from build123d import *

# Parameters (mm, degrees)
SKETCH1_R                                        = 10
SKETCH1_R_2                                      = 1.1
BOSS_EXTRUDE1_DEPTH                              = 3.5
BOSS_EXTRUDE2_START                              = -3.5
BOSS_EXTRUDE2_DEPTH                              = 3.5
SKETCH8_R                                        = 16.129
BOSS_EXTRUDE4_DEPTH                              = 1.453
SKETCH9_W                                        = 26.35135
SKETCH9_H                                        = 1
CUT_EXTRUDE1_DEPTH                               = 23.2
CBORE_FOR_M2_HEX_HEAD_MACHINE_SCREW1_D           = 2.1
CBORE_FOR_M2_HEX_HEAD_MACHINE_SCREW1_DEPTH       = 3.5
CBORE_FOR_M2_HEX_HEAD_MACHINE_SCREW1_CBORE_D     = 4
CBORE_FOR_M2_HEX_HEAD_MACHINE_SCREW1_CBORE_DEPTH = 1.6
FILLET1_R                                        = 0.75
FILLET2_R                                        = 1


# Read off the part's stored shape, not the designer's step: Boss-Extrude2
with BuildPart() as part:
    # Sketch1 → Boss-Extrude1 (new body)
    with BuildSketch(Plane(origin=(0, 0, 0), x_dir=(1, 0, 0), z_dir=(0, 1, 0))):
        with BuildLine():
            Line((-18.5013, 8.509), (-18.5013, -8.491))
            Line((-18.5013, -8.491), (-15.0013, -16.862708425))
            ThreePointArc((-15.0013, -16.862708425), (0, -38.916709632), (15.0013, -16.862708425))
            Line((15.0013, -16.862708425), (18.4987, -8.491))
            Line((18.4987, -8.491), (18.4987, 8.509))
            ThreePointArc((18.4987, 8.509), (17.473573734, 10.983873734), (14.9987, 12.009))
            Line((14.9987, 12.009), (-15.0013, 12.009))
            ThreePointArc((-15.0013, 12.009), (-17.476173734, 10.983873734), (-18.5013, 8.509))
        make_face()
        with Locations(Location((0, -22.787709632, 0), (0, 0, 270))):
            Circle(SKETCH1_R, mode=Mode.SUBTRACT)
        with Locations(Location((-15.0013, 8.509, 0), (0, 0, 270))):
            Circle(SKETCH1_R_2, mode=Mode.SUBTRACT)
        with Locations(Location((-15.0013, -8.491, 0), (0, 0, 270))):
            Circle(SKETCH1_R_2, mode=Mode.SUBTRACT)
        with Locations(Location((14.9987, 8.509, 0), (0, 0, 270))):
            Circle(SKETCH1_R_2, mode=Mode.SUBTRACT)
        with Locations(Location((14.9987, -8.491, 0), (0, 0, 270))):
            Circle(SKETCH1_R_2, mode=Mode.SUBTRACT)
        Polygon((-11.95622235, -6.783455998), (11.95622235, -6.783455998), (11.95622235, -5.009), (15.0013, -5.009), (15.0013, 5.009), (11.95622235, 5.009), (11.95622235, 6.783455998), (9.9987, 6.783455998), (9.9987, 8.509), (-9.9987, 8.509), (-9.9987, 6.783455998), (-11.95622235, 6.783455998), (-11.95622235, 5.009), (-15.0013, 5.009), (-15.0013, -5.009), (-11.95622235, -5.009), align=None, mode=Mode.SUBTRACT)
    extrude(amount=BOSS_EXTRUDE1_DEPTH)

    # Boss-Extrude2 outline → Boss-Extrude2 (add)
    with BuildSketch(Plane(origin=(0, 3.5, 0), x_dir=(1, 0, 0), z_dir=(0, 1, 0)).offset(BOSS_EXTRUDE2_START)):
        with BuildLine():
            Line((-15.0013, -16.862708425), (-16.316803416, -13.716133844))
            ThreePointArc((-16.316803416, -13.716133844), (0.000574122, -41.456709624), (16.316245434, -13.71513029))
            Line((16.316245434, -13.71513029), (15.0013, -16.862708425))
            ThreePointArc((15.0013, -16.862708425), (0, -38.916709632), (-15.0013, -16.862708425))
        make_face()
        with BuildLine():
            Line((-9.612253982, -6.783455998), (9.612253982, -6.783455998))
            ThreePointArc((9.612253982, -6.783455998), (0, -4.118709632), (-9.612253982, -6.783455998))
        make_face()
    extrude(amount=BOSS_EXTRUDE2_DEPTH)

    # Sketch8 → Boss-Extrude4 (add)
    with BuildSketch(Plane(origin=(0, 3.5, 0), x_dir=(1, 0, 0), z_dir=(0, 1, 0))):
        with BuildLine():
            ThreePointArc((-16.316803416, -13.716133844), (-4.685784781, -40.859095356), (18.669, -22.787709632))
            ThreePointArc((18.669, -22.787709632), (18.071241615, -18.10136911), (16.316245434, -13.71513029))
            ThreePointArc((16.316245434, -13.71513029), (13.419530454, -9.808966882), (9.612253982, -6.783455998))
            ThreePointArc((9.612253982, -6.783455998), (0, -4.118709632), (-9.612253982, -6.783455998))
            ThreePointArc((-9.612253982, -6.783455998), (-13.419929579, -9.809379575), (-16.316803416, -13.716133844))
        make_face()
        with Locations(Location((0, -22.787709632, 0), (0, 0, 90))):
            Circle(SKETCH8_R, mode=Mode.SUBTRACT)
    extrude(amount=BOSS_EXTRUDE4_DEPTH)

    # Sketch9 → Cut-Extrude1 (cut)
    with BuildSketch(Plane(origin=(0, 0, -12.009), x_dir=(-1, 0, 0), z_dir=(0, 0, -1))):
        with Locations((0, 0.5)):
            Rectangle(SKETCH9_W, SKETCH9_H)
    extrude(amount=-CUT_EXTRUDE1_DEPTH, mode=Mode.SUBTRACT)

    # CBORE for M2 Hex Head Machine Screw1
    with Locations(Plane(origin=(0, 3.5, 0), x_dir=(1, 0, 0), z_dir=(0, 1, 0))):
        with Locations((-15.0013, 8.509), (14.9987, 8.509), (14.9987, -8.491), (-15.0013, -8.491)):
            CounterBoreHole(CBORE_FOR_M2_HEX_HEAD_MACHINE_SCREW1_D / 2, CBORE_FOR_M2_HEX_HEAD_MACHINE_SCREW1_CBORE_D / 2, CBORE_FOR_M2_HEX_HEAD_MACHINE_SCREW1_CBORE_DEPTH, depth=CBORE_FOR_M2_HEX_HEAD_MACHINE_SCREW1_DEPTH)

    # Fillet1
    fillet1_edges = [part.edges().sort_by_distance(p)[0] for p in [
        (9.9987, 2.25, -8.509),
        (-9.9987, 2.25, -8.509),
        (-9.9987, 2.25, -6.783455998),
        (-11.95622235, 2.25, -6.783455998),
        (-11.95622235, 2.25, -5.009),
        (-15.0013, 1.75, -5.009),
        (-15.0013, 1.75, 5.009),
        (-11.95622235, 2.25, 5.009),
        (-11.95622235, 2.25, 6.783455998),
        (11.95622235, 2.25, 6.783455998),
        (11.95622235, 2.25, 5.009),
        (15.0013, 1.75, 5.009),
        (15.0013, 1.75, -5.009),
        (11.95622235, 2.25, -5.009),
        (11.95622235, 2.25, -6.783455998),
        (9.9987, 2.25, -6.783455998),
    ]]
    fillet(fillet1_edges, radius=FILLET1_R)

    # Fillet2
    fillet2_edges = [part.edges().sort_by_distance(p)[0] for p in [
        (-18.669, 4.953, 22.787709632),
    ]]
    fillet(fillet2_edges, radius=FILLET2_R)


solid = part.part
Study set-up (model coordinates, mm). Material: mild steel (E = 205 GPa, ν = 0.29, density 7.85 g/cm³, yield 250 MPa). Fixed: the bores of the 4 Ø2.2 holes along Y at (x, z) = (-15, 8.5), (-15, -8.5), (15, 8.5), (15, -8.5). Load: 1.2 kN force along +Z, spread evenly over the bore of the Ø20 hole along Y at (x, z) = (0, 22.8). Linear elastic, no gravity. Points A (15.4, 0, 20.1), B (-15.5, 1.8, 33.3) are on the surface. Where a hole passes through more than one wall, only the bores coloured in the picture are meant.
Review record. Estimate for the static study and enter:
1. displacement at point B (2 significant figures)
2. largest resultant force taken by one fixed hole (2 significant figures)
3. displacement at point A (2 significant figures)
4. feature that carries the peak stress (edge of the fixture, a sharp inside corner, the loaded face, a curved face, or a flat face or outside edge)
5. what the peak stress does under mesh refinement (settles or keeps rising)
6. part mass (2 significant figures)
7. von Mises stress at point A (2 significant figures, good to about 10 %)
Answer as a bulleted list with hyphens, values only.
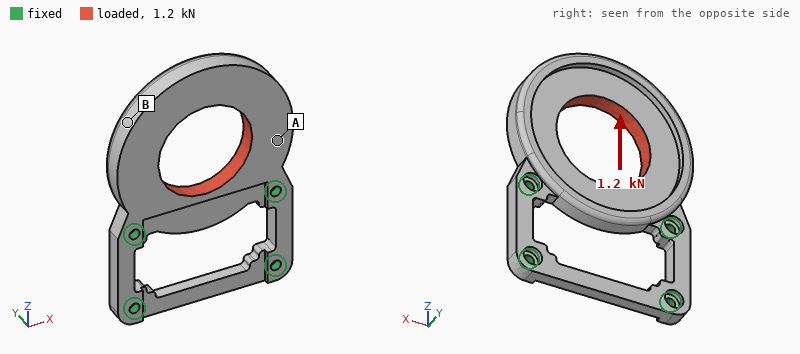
- 6.7 µm
- 590 N
- 3.7 µm
- edge of the fixture
- keeps rising
- 31 g
- 17 MPa
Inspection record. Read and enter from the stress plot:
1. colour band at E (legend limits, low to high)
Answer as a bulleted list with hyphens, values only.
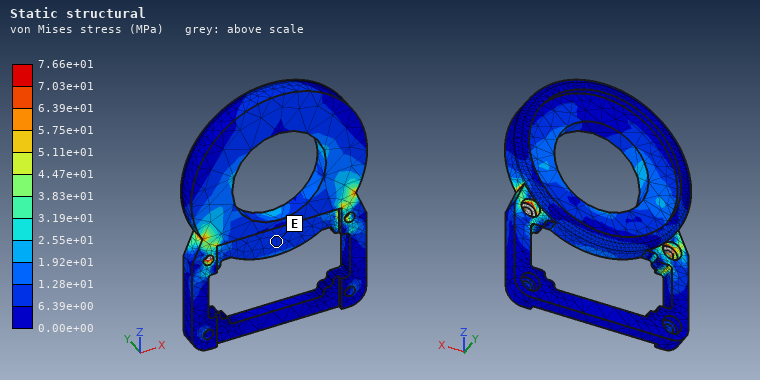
- 6.39e+00 to 1.28e+01 MPa
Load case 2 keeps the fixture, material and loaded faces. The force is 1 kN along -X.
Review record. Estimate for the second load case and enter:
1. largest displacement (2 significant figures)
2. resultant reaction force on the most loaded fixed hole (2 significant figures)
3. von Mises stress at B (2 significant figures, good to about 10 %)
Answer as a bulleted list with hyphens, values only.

- 13 µm
- 630 N
- 22 MPa
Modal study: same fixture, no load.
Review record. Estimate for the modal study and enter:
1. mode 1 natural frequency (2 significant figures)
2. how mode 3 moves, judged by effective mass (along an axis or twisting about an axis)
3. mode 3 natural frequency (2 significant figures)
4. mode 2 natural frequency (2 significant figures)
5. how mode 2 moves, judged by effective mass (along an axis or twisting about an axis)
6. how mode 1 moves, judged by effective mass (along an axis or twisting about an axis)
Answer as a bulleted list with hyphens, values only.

- 1900 Hz
- along X
- 9700 Hz
- 6000 Hz
- twisting about Z
- along Y
